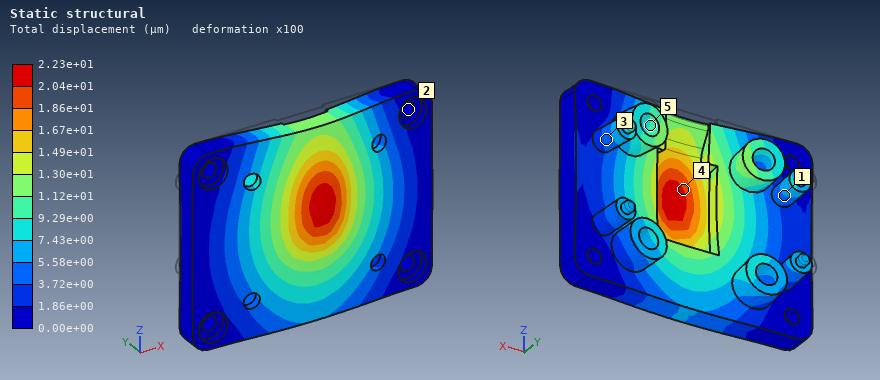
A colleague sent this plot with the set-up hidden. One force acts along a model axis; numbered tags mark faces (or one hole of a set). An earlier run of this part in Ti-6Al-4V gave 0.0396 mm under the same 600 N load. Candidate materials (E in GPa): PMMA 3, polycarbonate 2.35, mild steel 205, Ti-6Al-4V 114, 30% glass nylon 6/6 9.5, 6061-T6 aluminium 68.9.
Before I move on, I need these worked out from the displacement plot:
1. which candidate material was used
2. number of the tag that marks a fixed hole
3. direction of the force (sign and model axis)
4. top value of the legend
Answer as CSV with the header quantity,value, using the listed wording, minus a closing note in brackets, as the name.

quantity,value
which candidate material was used,mild steel
number of the tag that marks a fixed hole,2
direction of the force,-Y
top value of the legend,2.23e+01 µm
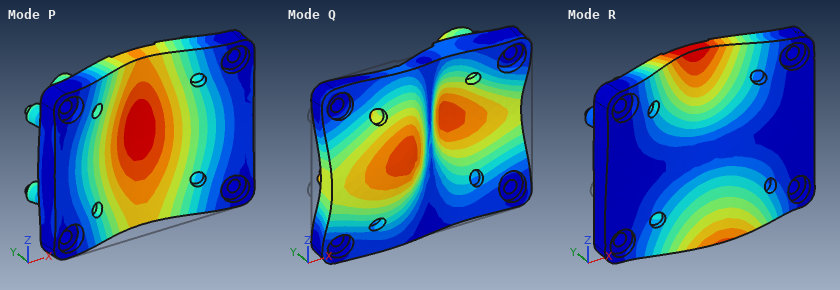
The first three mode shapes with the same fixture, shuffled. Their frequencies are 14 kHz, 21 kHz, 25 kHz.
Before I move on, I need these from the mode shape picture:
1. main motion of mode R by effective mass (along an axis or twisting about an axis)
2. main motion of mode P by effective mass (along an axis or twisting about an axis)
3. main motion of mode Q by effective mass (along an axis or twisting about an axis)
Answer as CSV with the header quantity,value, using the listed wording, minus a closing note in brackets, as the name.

quantity,value
main motion of mode R by effective mass,twisting about X
main motion of mode P by effective mass,along Y
main motion of mode Q by effective mass,twisting about Z
